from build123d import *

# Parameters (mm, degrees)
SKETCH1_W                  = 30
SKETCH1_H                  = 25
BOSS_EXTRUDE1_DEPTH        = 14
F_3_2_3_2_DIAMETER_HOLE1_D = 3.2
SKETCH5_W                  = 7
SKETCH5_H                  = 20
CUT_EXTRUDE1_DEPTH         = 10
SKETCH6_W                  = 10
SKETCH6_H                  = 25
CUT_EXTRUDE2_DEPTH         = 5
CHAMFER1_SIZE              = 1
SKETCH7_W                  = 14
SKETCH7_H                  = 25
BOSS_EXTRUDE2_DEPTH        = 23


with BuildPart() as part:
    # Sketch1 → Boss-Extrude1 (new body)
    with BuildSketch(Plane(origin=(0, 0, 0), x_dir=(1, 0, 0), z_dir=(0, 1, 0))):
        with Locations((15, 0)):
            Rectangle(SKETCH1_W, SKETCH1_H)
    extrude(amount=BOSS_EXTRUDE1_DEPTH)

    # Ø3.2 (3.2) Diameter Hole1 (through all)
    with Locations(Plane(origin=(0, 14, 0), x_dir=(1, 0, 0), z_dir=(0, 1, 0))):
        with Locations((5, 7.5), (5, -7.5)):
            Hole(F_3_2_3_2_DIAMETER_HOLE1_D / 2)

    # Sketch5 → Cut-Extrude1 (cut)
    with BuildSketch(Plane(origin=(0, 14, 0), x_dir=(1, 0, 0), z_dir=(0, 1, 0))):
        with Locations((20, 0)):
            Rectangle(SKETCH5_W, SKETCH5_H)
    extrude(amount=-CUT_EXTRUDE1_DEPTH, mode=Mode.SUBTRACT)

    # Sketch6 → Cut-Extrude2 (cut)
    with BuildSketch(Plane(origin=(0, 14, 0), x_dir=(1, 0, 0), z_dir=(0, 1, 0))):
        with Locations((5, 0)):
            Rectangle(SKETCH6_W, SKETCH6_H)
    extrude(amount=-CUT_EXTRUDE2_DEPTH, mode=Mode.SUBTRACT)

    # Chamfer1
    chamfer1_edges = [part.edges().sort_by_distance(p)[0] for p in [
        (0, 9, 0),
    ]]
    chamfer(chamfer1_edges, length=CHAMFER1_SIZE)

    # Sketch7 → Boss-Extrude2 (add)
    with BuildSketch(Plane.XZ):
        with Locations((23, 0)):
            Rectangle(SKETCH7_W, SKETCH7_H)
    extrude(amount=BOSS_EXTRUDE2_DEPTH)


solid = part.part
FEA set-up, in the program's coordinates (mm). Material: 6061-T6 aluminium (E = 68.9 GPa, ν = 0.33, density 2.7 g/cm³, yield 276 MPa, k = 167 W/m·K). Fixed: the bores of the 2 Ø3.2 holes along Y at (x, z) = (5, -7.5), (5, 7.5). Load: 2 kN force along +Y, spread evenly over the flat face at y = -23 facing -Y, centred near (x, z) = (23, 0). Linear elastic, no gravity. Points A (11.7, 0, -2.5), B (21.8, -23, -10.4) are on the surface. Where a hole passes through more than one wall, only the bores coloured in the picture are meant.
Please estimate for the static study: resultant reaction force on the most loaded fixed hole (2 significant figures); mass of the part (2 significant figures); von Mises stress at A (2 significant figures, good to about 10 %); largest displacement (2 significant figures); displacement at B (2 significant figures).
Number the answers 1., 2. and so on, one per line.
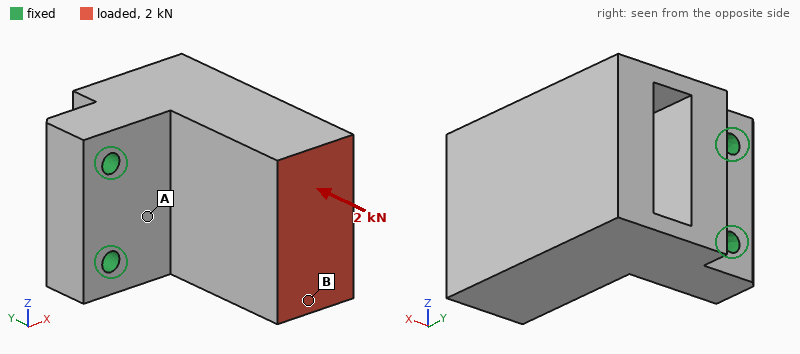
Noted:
1. 1.0 kN
2. 43 g
3. 51 MPa
4. 0.12 mm
5. 0.11 mm
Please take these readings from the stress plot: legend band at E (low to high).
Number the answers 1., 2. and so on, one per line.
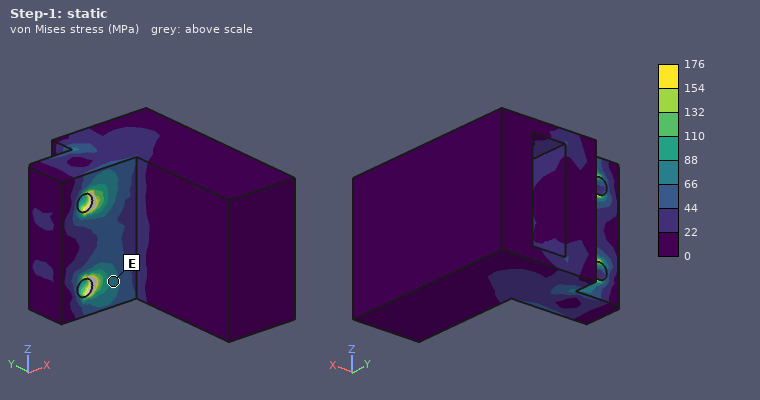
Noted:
1. 66 to 88 MPa
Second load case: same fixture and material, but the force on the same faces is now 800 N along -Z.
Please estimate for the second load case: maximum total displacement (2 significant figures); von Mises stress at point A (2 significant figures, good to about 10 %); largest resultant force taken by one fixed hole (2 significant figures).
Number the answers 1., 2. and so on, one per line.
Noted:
1. 52 µm
2. 42 MPa
3. 1.4 kN
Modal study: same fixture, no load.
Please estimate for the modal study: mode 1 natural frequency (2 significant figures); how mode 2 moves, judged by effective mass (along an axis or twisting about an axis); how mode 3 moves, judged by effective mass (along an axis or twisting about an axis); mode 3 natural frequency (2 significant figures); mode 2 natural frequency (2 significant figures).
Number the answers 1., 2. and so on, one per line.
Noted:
1. 3700 Hz
2. along Z
3. along Z
4. 11 kHz
5. 6300 Hz
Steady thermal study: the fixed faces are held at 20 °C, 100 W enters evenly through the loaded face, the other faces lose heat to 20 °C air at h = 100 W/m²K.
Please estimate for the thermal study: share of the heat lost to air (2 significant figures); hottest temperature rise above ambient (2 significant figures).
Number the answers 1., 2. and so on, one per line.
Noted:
1. 17 %
2. 78 K
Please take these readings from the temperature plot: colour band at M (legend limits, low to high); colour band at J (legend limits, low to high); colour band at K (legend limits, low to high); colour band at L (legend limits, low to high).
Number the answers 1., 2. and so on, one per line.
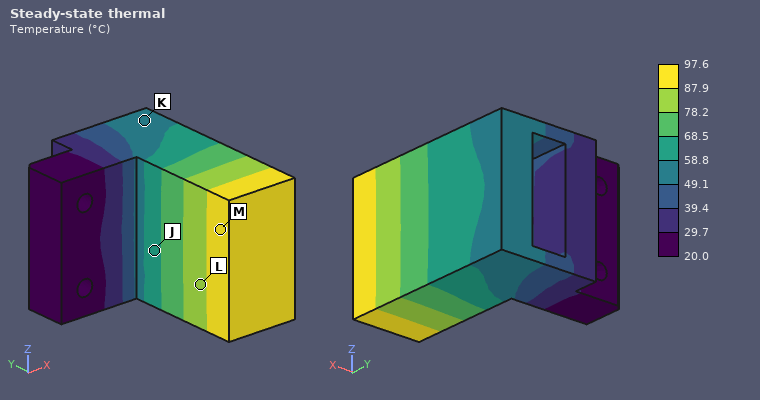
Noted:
1. 87.9 to 97.6 °C
2. 58.8 to 68.5 °C
3. 49.1 to 58.8 °C
4. 78.2 to 87.9 °C
